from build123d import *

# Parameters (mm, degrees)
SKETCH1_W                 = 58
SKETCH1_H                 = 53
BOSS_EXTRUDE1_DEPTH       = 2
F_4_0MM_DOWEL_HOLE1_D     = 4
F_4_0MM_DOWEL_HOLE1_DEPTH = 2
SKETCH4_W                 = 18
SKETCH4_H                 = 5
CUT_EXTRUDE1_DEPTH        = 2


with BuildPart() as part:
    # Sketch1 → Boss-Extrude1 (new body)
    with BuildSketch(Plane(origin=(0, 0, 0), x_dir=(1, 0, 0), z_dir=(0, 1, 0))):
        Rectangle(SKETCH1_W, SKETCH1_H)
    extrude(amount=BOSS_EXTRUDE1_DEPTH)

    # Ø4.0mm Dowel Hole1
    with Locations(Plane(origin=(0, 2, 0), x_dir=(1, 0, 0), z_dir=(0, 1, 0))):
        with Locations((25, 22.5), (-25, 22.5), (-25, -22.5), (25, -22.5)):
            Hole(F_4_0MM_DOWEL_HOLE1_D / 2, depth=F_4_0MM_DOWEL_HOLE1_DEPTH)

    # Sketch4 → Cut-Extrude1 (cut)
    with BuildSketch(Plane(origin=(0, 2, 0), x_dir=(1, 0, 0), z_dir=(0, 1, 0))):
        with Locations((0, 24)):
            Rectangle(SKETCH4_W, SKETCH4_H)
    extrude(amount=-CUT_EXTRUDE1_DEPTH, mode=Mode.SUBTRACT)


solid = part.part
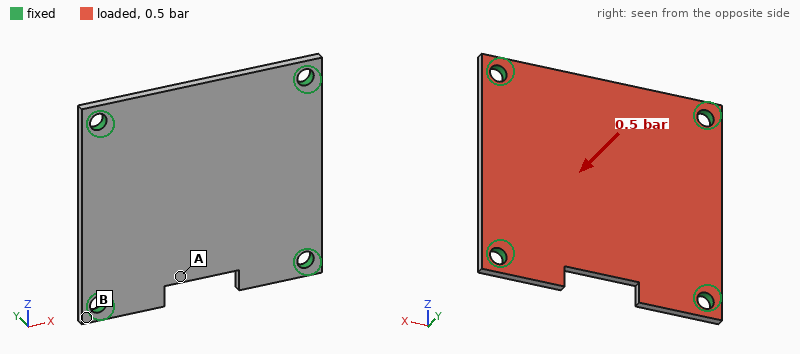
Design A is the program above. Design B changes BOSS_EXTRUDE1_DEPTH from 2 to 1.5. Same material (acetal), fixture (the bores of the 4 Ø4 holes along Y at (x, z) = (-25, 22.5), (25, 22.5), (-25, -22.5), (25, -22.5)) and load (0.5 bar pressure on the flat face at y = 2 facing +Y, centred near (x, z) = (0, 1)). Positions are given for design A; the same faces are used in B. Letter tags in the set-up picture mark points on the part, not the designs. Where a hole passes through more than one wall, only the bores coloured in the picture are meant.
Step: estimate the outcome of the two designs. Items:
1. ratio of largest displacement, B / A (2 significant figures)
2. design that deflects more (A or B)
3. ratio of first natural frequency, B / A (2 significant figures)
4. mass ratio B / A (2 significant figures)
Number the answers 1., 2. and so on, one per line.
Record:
1. 2.3
2. B
3. 0.76
4. 0.75
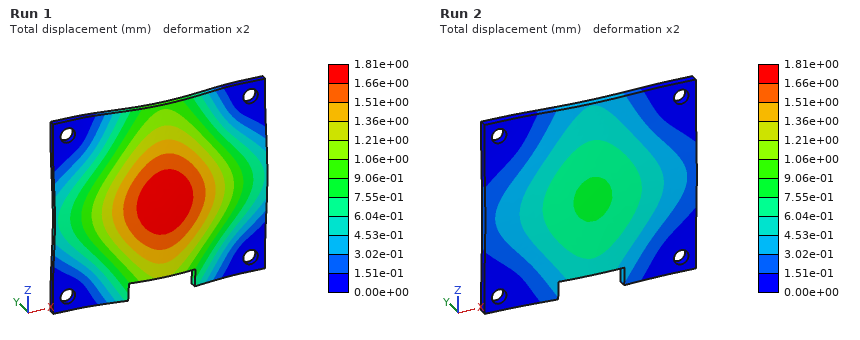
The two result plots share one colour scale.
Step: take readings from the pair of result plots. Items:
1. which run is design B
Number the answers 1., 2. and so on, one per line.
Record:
1. Run 1
